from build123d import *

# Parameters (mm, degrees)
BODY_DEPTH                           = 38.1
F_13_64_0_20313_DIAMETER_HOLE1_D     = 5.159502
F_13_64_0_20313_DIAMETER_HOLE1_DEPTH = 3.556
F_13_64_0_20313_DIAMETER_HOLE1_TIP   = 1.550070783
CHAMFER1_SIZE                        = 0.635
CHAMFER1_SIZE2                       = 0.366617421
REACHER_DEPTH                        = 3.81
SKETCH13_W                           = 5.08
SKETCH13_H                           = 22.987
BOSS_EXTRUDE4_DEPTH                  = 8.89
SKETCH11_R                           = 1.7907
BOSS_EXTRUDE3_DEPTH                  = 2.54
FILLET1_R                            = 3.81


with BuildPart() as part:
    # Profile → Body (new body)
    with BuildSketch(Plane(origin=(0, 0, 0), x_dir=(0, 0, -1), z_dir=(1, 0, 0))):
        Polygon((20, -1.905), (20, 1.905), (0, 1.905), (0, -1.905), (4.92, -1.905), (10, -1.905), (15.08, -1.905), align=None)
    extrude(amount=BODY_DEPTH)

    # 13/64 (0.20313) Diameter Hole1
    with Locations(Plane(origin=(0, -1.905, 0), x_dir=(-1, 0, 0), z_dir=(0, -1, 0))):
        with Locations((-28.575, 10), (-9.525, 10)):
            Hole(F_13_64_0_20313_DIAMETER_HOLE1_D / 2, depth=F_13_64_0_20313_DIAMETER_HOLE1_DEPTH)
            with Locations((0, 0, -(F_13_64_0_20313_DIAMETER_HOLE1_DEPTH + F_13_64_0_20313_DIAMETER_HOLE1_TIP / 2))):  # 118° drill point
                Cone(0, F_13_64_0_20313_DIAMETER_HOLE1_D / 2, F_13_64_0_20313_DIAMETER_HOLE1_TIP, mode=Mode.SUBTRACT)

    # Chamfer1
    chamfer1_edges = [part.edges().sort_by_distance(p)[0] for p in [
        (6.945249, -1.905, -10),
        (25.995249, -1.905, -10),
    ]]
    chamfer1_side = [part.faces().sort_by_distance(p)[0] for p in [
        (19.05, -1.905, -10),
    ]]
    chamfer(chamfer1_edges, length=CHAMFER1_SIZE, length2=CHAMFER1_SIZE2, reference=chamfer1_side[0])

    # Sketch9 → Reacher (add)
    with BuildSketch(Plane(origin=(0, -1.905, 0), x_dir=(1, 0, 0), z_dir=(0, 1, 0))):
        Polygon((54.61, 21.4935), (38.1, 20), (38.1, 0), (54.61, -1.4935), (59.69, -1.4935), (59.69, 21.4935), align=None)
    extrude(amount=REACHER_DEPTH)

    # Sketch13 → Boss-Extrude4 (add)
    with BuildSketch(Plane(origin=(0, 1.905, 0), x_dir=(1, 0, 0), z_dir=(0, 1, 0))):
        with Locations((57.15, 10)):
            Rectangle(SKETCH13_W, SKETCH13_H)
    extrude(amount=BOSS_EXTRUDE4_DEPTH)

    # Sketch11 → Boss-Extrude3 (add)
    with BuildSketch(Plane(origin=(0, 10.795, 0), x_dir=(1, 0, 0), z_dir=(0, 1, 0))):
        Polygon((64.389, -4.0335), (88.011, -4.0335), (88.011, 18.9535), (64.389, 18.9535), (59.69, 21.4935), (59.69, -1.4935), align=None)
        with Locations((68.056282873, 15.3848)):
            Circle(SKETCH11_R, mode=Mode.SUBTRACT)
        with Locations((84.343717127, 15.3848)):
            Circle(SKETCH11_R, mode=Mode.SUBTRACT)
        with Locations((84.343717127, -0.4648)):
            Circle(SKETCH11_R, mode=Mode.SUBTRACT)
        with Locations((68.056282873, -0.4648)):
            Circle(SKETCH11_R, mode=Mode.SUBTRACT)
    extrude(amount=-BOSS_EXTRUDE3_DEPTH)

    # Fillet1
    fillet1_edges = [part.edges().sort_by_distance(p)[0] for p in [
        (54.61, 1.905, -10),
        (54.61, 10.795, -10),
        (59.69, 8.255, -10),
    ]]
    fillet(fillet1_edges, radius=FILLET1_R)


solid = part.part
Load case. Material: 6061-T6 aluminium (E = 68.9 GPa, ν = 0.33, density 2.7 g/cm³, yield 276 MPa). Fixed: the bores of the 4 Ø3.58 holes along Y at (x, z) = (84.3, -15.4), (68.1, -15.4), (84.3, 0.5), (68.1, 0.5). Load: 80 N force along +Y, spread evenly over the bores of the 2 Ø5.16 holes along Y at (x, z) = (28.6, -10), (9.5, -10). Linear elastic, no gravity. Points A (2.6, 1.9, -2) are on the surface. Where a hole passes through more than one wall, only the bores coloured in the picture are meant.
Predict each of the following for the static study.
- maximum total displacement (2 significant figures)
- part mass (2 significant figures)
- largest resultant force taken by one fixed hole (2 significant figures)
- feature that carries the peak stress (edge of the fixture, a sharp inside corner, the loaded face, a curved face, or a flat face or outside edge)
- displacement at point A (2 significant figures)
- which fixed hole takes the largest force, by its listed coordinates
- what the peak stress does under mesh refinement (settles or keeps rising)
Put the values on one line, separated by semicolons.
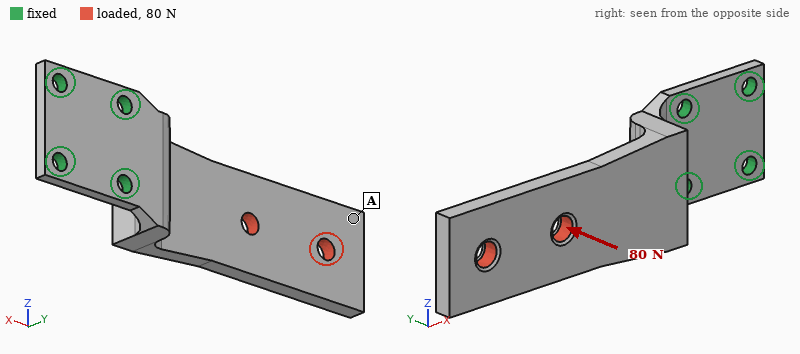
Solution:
1.1 mm; 19 g; 67 N; edge of the fixture; 1.0 mm; (68.1, -15.4); keeps rising
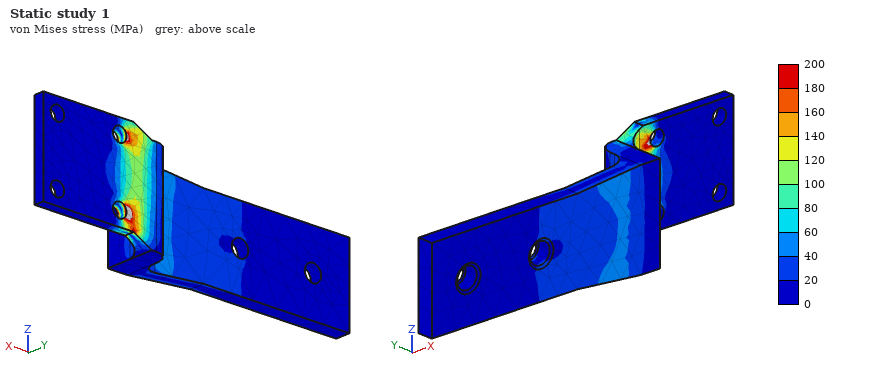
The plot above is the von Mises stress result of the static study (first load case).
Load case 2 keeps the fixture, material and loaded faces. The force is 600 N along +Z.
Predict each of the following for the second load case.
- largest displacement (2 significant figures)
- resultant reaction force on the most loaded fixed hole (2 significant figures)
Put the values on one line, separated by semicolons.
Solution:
0.44 mm; 1.8 kN
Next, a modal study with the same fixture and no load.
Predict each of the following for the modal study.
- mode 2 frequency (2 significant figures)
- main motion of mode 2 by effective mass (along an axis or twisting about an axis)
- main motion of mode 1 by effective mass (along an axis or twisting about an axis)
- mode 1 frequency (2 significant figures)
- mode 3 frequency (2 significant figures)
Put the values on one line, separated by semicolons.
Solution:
2500 Hz; along Z; along Y; 570 Hz; 3100 Hz
